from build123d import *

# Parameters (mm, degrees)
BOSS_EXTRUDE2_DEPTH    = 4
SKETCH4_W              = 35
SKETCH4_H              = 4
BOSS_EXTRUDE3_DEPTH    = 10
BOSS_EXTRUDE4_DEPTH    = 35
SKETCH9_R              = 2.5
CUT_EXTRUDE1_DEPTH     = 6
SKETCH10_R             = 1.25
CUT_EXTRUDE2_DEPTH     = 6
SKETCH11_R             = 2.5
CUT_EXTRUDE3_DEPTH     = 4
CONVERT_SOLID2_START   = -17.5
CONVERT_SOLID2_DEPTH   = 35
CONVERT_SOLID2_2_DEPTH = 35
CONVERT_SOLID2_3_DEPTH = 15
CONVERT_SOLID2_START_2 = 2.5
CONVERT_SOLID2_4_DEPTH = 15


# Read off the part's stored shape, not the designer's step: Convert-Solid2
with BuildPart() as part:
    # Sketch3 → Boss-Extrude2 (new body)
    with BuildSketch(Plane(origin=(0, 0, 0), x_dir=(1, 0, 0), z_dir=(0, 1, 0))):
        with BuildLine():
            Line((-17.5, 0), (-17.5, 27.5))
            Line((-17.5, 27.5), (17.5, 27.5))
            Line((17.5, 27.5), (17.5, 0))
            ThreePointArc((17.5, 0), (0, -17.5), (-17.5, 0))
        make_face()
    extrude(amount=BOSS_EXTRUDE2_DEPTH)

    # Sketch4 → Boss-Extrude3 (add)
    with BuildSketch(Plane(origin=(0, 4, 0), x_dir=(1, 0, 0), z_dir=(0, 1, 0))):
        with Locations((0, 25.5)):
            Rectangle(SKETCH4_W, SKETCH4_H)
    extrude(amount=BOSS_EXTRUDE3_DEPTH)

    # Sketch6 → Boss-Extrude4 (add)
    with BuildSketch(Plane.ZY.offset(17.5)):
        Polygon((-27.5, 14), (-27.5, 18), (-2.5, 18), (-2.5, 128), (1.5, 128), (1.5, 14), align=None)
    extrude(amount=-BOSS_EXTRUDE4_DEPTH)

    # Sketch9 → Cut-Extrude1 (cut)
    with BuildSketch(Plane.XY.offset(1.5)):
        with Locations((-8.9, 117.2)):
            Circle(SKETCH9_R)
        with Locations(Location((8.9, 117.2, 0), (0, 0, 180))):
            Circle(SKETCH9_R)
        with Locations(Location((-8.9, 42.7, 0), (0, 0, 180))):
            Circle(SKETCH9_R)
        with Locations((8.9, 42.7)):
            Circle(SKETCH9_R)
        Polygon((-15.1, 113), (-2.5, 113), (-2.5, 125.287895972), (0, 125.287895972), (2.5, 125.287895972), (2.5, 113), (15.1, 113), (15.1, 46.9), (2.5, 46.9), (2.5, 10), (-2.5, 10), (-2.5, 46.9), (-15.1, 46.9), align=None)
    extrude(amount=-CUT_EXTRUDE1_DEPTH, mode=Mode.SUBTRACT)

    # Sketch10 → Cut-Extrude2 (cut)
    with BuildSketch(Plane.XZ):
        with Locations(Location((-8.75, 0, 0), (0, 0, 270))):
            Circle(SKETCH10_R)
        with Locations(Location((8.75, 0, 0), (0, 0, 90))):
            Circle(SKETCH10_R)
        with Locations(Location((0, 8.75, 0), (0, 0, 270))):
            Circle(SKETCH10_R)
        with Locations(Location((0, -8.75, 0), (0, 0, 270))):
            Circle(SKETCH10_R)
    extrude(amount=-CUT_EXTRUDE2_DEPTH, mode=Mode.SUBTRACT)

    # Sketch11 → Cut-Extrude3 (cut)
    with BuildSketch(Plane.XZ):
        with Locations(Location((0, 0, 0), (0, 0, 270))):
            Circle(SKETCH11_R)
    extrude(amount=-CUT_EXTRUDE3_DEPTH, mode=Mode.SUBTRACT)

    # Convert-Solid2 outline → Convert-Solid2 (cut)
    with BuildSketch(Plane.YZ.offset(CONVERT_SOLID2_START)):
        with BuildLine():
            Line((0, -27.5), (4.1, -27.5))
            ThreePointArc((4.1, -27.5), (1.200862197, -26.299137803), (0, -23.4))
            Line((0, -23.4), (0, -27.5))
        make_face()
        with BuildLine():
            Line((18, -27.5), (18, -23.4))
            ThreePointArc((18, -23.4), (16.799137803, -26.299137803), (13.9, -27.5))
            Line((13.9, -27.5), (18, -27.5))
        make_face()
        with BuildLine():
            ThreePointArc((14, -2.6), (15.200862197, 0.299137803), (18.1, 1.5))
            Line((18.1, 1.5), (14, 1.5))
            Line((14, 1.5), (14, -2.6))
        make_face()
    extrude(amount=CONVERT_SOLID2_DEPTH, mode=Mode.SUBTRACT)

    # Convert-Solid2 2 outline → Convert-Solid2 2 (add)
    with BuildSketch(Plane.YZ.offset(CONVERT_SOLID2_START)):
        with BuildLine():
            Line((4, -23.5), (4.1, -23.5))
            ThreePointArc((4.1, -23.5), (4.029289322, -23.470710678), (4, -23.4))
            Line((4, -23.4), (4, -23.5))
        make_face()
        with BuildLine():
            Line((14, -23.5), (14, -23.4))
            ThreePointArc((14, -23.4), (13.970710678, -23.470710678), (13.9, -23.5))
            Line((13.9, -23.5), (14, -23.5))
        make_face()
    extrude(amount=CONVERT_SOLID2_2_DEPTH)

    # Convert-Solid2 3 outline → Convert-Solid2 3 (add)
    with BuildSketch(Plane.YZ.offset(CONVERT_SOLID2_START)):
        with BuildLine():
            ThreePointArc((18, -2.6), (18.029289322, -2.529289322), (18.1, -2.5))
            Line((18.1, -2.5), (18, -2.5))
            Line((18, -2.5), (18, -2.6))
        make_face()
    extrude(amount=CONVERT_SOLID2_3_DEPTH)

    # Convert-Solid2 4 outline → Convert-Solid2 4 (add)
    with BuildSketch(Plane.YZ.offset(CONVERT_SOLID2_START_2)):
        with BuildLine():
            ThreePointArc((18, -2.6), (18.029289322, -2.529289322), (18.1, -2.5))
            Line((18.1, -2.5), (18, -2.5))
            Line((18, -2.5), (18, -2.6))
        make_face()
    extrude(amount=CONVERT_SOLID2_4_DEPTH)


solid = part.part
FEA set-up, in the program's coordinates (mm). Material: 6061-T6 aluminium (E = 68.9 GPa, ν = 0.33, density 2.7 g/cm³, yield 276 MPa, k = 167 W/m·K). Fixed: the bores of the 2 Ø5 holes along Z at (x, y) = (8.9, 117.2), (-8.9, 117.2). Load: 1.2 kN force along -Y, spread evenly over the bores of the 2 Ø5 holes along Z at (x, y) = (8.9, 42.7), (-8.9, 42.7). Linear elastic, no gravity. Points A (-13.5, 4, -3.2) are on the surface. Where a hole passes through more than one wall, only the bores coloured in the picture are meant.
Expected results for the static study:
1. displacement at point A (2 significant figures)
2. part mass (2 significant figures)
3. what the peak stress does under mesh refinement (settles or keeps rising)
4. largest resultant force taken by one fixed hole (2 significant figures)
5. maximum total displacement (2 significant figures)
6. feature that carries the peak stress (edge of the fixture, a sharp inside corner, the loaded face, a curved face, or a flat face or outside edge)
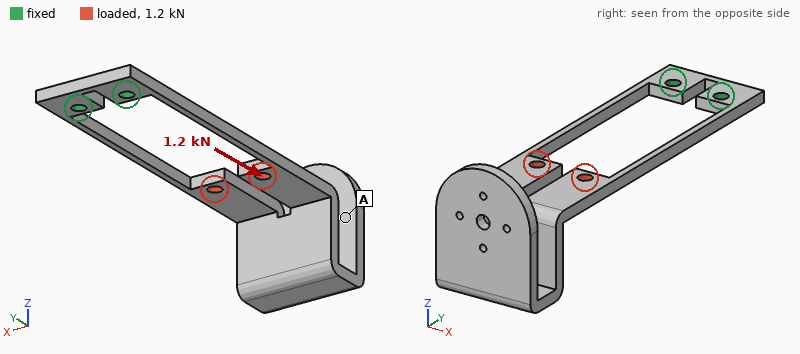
0.12 mm
46 g
keeps rising
630 N
0.30 mm
a sharp inside corner
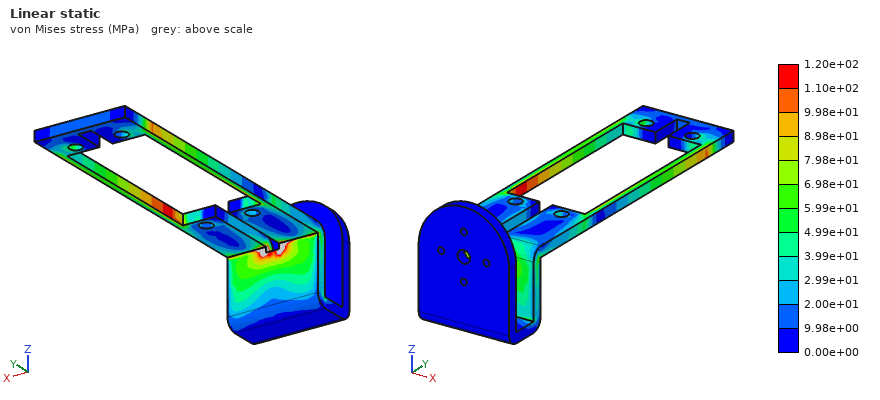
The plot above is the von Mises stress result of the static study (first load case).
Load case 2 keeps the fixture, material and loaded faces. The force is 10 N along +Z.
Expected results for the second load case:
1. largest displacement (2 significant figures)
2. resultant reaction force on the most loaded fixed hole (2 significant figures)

1.4 mm
5.0 N
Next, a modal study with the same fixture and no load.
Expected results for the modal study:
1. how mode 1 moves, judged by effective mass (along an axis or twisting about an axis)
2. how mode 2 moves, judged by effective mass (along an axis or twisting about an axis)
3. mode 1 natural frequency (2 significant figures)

along Z
along X
56 Hz
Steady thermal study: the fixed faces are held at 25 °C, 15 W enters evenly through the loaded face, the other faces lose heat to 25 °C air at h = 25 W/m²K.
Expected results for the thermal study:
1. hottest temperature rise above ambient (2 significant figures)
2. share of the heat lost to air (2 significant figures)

71 K
83 %
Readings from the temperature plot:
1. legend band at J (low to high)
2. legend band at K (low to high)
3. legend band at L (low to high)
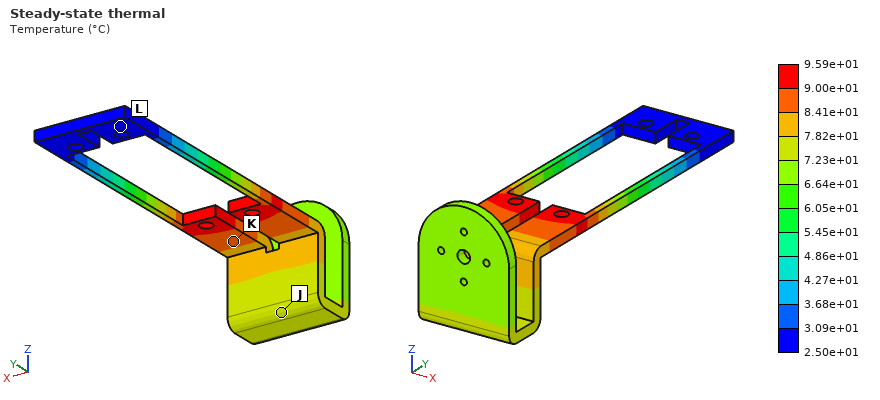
7.23e+01 to 7.82e+01 °C
8.41e+01 to 9.00e+01 °C
2.50e+01 to 3.09e+01 °C
